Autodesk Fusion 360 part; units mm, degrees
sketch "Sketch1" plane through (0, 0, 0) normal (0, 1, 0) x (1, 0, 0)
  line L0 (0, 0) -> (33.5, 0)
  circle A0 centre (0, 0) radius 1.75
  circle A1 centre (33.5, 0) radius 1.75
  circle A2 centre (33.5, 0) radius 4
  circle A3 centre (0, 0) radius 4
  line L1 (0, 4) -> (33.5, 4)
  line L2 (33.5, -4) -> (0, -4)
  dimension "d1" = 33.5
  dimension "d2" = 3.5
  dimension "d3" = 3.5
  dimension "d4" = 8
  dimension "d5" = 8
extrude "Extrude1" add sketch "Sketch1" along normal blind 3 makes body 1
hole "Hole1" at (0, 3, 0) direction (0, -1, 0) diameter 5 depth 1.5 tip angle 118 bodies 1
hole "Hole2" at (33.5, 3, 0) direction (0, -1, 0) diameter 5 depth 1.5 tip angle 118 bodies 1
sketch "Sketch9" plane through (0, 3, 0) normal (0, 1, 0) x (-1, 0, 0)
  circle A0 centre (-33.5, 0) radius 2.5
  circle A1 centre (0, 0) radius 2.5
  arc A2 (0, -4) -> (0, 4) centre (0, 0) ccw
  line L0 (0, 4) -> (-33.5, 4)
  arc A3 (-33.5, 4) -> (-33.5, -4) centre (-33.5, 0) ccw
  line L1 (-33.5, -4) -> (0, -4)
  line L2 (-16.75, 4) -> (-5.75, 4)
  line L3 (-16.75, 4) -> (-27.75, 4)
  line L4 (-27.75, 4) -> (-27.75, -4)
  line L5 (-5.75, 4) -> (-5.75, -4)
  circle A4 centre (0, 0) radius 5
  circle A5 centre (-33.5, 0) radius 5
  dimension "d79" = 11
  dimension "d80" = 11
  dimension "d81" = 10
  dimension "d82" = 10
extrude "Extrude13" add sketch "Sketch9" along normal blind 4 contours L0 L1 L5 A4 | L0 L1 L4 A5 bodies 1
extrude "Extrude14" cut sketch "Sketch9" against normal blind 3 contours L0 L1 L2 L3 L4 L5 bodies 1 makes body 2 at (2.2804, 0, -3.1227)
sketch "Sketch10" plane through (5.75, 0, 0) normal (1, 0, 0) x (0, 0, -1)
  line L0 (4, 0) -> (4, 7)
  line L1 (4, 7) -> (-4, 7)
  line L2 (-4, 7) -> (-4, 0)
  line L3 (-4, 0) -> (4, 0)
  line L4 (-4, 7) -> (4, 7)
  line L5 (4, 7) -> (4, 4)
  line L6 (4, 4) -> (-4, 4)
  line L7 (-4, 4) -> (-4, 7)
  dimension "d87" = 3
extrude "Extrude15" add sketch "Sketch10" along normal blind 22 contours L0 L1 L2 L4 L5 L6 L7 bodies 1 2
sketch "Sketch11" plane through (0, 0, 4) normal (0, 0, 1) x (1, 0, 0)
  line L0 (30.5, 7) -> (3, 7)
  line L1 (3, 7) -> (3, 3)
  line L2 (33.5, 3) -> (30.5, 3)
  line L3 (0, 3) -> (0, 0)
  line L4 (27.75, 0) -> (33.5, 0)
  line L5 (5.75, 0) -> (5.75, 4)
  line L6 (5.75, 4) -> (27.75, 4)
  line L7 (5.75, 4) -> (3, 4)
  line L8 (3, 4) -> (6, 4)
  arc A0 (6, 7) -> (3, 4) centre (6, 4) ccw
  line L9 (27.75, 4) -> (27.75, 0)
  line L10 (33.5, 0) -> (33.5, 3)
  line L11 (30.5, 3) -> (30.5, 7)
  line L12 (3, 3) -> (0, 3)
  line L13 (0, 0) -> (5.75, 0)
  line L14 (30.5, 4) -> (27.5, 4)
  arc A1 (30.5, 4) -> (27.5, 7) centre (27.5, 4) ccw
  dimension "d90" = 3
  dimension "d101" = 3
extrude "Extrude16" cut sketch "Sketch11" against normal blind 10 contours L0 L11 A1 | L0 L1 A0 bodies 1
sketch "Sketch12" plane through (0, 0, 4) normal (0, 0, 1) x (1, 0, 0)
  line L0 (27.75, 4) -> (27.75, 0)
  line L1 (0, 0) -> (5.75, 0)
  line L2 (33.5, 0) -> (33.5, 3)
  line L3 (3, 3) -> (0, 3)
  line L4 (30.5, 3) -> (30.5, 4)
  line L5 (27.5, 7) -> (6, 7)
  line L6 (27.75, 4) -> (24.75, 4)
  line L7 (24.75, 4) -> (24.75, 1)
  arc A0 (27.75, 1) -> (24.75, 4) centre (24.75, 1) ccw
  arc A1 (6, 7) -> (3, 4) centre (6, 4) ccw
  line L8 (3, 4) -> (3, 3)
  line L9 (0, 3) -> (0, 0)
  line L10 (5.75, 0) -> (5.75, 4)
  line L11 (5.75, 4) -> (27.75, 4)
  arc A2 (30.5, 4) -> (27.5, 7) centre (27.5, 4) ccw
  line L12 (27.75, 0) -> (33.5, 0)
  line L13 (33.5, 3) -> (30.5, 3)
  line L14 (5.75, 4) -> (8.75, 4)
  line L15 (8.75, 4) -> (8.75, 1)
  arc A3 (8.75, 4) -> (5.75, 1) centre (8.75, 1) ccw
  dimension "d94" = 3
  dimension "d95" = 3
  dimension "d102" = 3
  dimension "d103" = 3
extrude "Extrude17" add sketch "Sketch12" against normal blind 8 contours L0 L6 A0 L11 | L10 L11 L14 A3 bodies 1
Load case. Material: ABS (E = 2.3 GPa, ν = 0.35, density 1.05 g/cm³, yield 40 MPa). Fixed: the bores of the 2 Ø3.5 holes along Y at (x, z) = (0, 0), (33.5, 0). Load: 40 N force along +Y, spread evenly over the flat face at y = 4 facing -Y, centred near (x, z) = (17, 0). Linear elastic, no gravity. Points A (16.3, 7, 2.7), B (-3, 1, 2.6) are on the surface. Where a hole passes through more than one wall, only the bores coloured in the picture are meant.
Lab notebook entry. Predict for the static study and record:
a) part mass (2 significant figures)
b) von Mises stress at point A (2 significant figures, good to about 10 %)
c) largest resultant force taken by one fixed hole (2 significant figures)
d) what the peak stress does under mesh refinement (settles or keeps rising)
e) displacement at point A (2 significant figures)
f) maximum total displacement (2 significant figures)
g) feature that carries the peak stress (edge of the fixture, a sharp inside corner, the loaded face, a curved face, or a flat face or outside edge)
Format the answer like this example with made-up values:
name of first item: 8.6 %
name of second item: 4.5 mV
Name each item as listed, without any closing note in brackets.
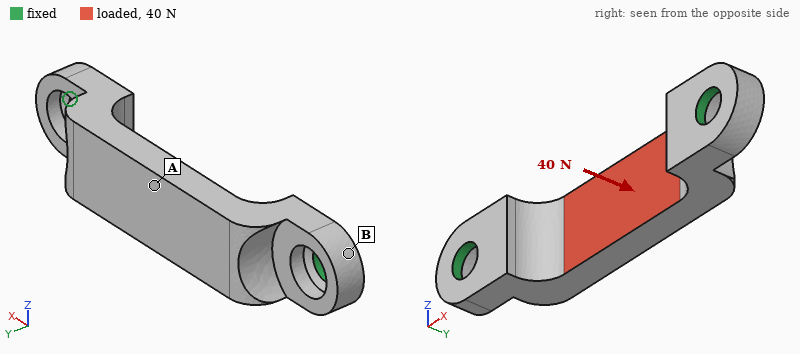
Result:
part mass: 1.0 g
von Mises stress at point A: 5.9 MPa
largest resultant force taken by one fixed hole: 39 N
what the peak stress does under mesh refinement: keeps rising
displacement at point A: 66 µm
maximum total displacement: 69 µm
feature that carries the peak stress: edge of the fixture
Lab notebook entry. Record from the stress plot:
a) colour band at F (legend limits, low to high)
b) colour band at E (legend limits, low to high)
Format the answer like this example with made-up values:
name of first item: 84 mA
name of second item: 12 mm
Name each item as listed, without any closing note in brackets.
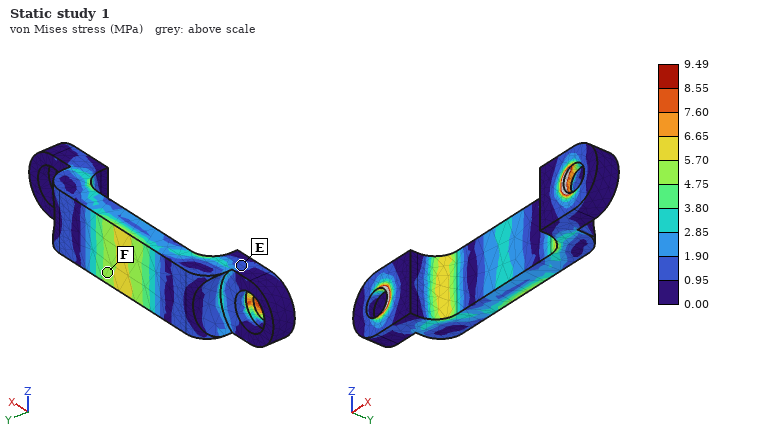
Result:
colour band at F: 4.75 to 5.70 MPa
colour band at E: 0.95 to 1.90 MPa
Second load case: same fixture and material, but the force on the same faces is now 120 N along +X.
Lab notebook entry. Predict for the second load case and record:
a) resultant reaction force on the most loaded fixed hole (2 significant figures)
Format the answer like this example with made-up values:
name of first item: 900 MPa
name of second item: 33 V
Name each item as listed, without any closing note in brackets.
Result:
resultant reaction force on the most loaded fixed hole: 61 N
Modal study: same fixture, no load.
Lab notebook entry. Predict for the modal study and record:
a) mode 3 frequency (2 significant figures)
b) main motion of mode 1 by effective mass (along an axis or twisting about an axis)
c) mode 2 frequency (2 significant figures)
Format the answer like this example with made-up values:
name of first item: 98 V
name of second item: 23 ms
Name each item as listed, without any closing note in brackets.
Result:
mode 3 frequency: 6400 Hz
main motion of mode 1 by effective mass: along Z
mode 2 frequency: 6300 Hz
